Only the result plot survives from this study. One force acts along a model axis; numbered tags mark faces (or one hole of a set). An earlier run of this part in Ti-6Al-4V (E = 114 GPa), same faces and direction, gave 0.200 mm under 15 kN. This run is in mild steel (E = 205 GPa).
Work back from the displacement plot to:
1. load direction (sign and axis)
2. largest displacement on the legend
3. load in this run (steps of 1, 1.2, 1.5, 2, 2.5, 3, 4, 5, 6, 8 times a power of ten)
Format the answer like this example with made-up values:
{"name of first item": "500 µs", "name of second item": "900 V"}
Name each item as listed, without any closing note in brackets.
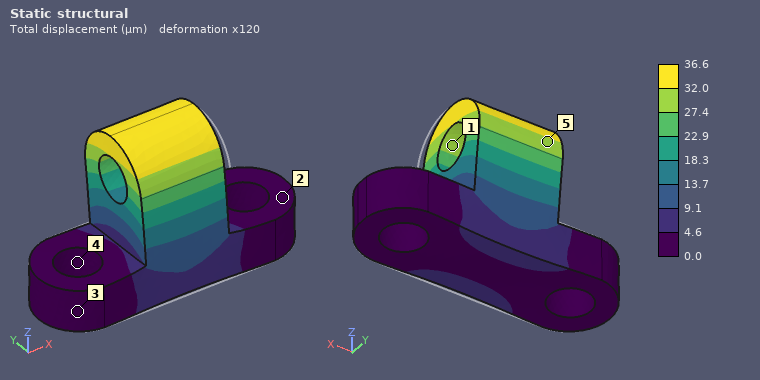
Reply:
{"load direction": "+Y", "largest displacement on the legend": "36.6 µm", "load in this run": "5 kN"}
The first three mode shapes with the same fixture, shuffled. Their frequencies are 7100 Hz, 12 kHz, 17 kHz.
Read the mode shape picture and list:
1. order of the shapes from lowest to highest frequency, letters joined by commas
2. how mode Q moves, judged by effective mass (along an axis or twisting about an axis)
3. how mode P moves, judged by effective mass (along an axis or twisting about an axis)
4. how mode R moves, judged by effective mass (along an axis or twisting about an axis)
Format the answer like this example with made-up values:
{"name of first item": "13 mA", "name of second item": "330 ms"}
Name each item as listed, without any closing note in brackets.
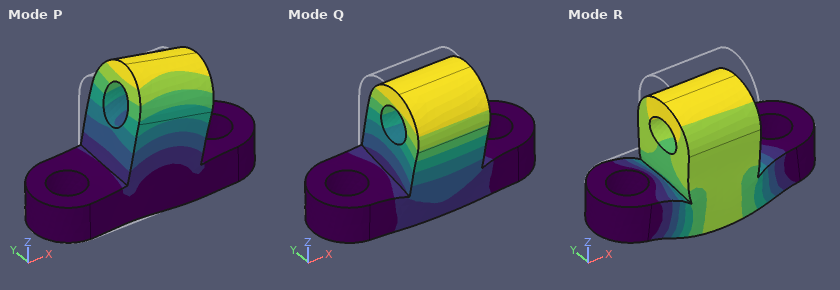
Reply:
{"order of the shapes from lowest to highest frequency, letters joined by commas": "Q, P, R", "how mode Q moves, judged by effective mass": "along Y", "how mode P moves, judged by effective mass": "along X", "how mode R moves, judged by effective mass": "along Z"}
